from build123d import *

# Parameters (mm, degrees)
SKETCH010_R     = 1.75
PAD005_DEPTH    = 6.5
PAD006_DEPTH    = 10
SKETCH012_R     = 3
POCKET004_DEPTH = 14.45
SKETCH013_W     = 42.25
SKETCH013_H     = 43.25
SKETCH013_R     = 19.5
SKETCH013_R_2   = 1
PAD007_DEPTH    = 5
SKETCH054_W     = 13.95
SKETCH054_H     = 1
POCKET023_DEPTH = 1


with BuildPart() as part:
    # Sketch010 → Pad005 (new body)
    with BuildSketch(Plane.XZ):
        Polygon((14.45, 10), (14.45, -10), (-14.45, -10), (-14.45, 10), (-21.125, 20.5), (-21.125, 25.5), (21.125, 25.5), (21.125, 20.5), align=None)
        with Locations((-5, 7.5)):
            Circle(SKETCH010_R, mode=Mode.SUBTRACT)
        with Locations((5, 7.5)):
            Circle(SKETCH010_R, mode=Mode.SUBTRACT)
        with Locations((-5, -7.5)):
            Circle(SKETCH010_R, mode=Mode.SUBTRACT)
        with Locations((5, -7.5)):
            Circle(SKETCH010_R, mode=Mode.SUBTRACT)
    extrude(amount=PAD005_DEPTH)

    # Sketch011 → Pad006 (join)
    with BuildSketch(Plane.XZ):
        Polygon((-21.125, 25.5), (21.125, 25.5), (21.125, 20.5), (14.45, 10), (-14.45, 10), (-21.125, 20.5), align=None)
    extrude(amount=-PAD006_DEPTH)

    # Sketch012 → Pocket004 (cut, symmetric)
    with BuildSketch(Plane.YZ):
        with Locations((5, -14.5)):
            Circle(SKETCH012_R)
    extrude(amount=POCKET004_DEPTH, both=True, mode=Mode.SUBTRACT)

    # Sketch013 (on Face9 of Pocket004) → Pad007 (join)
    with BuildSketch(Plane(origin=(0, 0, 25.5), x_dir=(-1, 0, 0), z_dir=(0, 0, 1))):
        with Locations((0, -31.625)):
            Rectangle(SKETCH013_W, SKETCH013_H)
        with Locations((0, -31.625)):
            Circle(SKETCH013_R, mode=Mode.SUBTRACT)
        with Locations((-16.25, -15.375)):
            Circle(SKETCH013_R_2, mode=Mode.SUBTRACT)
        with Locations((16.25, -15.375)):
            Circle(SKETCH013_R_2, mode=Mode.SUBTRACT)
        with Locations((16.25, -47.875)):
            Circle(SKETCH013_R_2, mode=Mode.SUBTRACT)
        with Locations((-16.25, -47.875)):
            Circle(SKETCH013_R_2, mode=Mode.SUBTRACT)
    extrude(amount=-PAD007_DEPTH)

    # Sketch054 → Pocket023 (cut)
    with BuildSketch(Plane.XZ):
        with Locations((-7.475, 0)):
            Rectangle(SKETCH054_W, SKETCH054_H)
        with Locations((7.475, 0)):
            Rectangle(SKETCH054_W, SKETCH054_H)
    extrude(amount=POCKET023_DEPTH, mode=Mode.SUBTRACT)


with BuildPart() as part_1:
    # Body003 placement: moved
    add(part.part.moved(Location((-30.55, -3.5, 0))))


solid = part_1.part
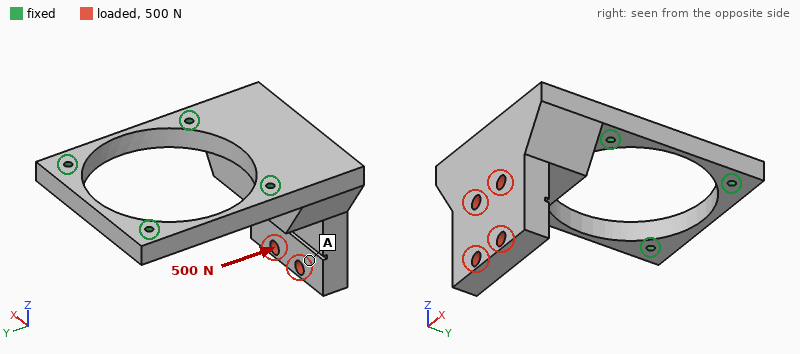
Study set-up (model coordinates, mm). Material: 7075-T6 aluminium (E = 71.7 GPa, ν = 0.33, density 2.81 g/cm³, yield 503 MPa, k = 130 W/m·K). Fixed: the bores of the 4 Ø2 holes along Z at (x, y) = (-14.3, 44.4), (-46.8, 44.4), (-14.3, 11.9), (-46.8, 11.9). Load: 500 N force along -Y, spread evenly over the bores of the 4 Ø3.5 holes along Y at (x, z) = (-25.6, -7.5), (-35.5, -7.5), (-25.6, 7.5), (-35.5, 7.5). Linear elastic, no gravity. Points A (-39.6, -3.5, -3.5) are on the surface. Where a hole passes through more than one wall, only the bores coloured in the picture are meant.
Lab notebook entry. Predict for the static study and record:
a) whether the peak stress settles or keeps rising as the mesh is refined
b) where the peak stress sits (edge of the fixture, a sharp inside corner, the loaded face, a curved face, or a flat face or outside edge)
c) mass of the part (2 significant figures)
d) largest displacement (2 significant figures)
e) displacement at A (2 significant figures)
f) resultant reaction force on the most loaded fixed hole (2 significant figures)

keeps rising
edge of the fixture
46 g
0.25 mm
0.19 mm
270 N
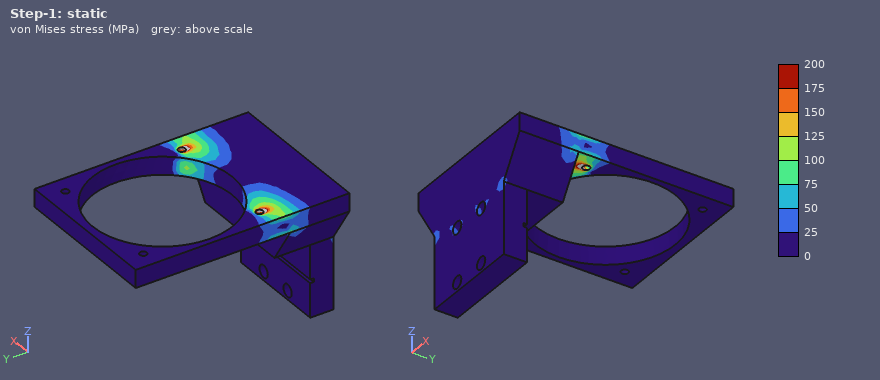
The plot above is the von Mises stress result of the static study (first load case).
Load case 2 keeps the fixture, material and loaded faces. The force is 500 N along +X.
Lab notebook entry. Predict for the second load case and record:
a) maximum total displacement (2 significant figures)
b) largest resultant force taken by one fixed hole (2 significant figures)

20 µm
500 N
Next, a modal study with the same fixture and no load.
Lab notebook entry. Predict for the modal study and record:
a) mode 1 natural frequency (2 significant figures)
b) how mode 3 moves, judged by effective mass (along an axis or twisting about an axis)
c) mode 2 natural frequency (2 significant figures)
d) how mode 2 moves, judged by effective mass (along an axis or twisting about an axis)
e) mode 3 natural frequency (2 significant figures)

1900 Hz
along Z
7700 Hz
along X
9600 Hz
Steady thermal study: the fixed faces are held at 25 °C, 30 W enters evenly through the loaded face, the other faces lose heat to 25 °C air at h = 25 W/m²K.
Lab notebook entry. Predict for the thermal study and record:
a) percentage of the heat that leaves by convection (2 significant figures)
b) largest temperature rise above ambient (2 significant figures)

9.1 %
42 K
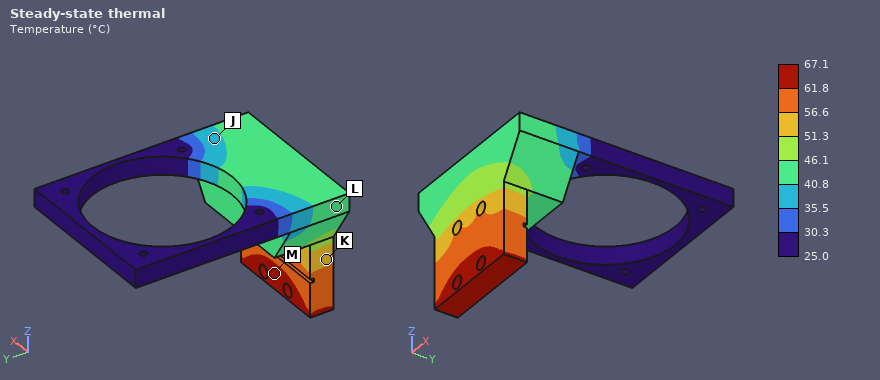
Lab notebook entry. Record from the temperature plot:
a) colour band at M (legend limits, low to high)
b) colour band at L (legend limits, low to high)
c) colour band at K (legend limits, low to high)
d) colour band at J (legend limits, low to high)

61.8 to 67.1 °C
40.8 to 46.1 °C
51.3 to 56.6 °C
35.5 to 40.8 °C
